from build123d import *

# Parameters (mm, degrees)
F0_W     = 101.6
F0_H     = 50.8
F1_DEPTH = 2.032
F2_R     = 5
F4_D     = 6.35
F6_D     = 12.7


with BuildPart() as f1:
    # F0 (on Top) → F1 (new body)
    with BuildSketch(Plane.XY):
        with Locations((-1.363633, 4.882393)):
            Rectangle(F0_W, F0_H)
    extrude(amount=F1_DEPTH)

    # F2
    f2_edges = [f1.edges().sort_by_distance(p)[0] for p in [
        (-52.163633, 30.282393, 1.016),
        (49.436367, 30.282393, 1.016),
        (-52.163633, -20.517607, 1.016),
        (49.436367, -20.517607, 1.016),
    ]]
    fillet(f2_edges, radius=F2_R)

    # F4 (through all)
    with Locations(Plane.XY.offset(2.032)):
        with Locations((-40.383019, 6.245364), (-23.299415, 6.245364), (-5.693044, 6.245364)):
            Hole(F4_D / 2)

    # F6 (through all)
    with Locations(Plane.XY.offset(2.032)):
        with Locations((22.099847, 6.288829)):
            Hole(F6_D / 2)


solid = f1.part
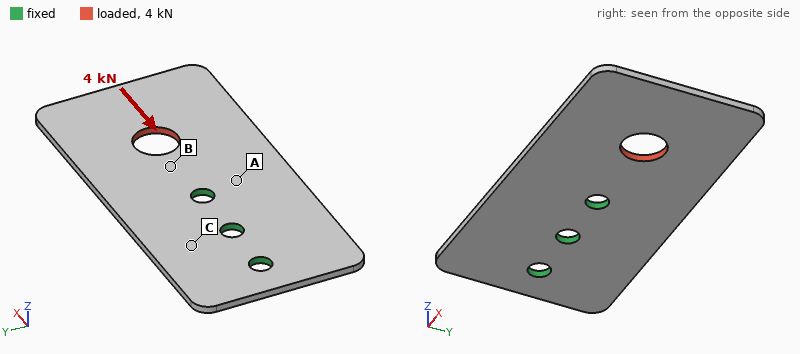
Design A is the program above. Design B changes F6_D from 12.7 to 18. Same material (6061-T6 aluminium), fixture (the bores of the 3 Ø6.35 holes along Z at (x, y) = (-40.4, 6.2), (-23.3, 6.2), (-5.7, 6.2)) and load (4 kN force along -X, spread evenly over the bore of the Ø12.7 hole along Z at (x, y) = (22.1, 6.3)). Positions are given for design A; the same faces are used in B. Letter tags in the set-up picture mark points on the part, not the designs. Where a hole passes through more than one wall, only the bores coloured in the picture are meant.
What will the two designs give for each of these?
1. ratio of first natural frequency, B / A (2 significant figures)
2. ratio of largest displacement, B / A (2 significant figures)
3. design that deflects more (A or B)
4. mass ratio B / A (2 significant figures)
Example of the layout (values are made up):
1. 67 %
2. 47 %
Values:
1. 0.98
2. 1.1
3. B
4. 0.97
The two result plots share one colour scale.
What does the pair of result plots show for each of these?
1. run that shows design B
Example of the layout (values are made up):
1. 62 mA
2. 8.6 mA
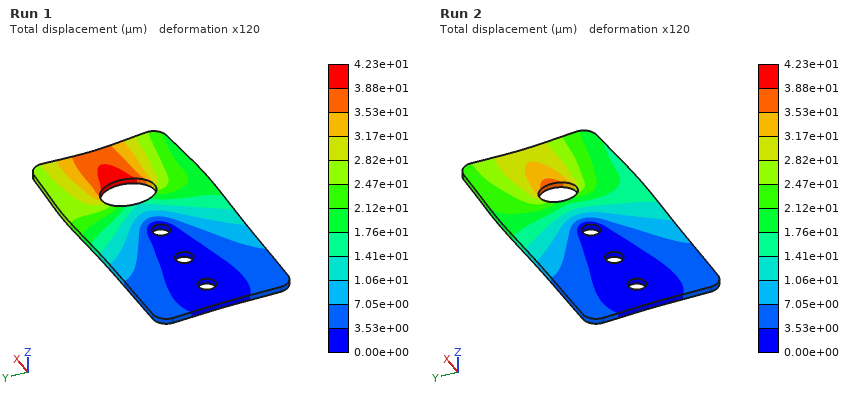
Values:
1. Run 1
